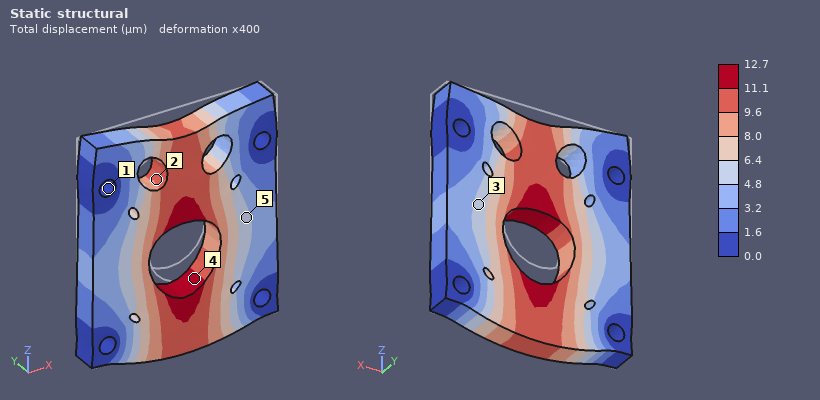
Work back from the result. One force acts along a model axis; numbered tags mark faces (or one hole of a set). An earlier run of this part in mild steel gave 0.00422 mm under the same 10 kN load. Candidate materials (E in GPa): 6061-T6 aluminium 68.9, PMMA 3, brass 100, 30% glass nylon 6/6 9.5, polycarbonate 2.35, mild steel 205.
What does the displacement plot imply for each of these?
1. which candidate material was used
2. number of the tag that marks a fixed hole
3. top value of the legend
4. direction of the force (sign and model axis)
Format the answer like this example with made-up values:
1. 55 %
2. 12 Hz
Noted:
1. 6061-T6 aluminium
2. 1
3. 12.7 µm
4. -Z
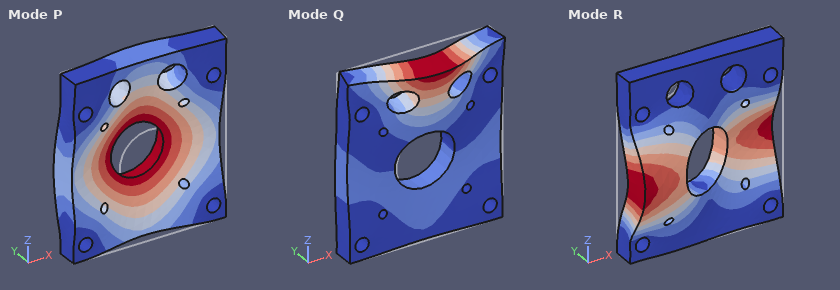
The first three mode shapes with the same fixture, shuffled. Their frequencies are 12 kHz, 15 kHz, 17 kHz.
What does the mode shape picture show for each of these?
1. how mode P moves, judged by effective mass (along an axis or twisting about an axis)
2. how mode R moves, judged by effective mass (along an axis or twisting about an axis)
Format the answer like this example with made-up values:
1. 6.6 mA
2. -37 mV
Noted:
1. along Y
2. twisting about Z
